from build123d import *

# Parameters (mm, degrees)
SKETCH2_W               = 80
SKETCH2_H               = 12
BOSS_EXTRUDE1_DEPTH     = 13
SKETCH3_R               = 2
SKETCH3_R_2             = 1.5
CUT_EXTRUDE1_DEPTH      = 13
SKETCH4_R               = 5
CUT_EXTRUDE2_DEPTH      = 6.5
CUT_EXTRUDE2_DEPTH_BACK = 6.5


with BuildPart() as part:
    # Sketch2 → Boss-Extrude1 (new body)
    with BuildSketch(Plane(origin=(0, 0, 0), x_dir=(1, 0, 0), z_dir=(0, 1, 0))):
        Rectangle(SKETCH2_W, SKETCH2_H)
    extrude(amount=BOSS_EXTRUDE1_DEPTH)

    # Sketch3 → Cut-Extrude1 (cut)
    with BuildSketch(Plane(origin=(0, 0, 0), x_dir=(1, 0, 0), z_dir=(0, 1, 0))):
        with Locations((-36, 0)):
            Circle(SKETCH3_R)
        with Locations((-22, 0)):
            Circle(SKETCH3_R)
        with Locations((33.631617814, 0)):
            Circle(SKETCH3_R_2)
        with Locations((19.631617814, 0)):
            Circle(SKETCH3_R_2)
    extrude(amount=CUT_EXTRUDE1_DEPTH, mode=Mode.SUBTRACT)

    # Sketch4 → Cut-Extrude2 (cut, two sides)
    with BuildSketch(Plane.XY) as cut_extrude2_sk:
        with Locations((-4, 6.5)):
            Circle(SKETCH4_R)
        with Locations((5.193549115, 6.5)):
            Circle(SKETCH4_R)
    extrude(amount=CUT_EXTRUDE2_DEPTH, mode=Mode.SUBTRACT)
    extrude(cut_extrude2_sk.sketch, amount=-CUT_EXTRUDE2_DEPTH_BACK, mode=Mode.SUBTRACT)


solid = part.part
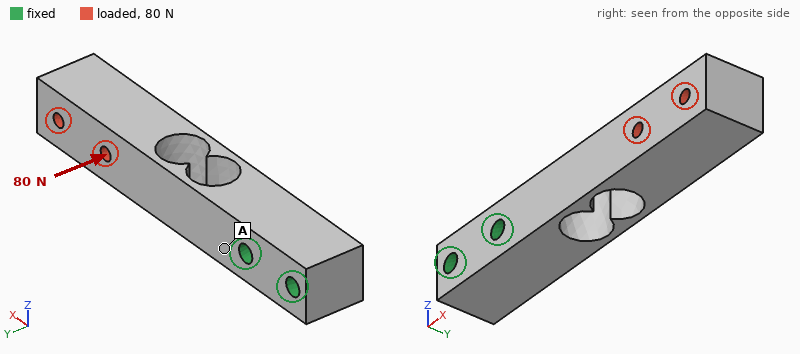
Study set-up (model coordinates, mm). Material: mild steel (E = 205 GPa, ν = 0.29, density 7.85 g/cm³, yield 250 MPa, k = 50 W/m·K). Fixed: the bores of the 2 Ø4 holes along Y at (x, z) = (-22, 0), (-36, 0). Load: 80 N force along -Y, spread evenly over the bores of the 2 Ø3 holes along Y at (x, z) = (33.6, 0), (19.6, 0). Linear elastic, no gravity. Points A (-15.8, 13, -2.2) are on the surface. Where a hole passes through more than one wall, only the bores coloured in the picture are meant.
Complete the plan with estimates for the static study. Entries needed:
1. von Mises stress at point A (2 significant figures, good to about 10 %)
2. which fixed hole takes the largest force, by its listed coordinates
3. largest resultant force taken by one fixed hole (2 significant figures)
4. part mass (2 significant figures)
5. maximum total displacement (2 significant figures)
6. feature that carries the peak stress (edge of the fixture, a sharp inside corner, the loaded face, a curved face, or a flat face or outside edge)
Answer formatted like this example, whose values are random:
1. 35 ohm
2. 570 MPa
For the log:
1. 11 MPa
2. (-22, 0)
3. 110 N
4. 79 g
5. 26 µm
6. a curved face
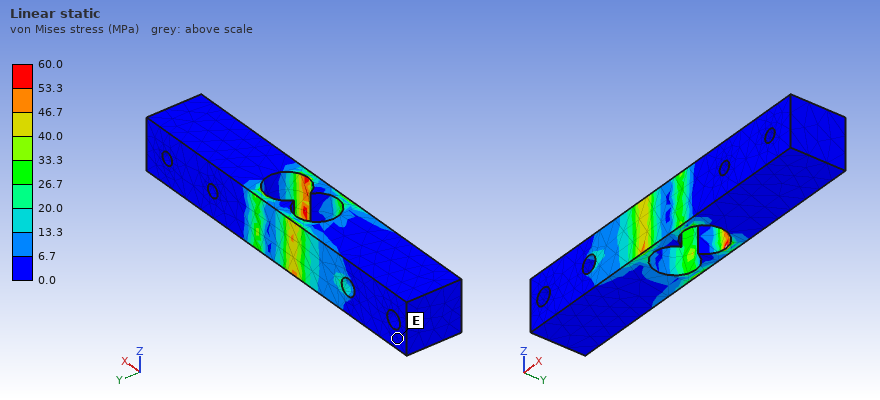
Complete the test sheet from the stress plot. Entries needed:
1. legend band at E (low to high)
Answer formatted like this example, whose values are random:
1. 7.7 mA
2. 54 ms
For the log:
1. 0.0 to 6.7 MPa
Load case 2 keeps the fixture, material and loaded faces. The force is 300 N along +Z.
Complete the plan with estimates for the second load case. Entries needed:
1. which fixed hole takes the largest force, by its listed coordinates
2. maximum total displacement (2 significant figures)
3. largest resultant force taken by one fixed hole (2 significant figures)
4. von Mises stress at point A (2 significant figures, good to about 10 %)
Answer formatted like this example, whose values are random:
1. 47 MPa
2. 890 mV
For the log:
1. (-22, 0)
2. 0.10 mm
3. 770 N
4. 18 MPa
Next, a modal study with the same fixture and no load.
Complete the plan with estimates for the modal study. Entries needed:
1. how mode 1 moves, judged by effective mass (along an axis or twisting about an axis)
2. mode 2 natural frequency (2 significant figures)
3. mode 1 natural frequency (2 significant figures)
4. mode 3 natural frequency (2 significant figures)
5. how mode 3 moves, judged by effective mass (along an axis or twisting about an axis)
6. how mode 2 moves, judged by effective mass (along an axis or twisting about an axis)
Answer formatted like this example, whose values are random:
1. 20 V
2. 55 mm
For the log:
1. along Y
2. 1700 Hz
3. 1600 Hz
4. 6800 Hz
5. twisting about X
6. along Z
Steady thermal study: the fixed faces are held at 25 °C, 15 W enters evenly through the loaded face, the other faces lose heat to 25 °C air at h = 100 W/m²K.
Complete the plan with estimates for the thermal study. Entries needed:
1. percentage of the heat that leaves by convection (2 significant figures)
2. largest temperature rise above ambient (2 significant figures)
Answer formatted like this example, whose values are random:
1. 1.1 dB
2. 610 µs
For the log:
1. 78 %
2. 59 K
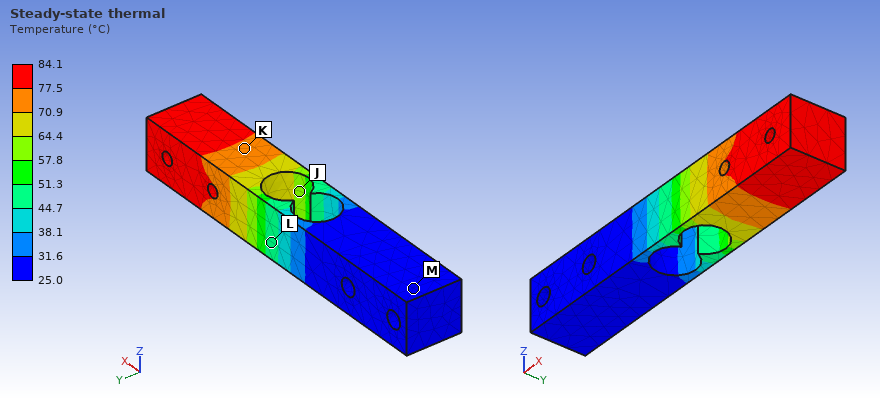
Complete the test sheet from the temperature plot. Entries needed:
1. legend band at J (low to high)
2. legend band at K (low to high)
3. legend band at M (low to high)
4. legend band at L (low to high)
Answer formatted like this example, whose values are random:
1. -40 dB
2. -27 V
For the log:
1. 57.8 to 64.4 °C
2. 70.9 to 77.5 °C
3. 25.0 to 31.6 °C
4. 44.7 to 51.3 °C
